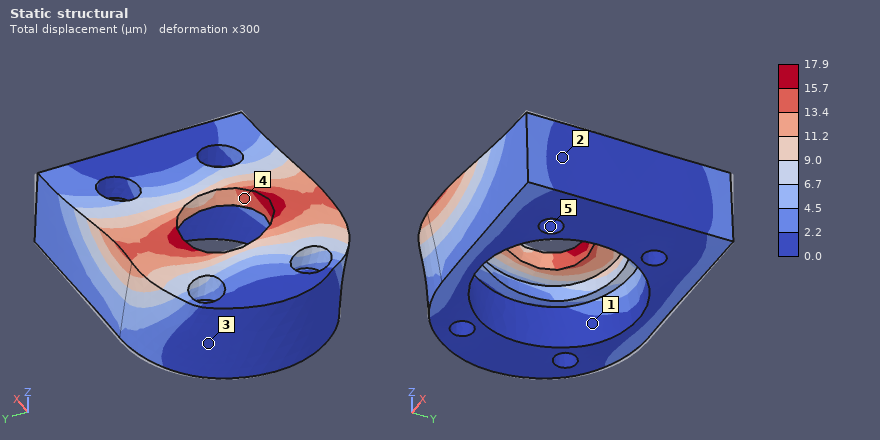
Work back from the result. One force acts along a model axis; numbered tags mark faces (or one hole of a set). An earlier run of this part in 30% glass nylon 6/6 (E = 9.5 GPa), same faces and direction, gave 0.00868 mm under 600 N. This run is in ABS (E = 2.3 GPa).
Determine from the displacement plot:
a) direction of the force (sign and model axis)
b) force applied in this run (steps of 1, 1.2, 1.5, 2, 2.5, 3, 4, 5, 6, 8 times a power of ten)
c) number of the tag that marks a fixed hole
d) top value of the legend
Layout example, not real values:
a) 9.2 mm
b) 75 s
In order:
a) -Y
b) 300 N
c) 5
d) 17.9 µm
